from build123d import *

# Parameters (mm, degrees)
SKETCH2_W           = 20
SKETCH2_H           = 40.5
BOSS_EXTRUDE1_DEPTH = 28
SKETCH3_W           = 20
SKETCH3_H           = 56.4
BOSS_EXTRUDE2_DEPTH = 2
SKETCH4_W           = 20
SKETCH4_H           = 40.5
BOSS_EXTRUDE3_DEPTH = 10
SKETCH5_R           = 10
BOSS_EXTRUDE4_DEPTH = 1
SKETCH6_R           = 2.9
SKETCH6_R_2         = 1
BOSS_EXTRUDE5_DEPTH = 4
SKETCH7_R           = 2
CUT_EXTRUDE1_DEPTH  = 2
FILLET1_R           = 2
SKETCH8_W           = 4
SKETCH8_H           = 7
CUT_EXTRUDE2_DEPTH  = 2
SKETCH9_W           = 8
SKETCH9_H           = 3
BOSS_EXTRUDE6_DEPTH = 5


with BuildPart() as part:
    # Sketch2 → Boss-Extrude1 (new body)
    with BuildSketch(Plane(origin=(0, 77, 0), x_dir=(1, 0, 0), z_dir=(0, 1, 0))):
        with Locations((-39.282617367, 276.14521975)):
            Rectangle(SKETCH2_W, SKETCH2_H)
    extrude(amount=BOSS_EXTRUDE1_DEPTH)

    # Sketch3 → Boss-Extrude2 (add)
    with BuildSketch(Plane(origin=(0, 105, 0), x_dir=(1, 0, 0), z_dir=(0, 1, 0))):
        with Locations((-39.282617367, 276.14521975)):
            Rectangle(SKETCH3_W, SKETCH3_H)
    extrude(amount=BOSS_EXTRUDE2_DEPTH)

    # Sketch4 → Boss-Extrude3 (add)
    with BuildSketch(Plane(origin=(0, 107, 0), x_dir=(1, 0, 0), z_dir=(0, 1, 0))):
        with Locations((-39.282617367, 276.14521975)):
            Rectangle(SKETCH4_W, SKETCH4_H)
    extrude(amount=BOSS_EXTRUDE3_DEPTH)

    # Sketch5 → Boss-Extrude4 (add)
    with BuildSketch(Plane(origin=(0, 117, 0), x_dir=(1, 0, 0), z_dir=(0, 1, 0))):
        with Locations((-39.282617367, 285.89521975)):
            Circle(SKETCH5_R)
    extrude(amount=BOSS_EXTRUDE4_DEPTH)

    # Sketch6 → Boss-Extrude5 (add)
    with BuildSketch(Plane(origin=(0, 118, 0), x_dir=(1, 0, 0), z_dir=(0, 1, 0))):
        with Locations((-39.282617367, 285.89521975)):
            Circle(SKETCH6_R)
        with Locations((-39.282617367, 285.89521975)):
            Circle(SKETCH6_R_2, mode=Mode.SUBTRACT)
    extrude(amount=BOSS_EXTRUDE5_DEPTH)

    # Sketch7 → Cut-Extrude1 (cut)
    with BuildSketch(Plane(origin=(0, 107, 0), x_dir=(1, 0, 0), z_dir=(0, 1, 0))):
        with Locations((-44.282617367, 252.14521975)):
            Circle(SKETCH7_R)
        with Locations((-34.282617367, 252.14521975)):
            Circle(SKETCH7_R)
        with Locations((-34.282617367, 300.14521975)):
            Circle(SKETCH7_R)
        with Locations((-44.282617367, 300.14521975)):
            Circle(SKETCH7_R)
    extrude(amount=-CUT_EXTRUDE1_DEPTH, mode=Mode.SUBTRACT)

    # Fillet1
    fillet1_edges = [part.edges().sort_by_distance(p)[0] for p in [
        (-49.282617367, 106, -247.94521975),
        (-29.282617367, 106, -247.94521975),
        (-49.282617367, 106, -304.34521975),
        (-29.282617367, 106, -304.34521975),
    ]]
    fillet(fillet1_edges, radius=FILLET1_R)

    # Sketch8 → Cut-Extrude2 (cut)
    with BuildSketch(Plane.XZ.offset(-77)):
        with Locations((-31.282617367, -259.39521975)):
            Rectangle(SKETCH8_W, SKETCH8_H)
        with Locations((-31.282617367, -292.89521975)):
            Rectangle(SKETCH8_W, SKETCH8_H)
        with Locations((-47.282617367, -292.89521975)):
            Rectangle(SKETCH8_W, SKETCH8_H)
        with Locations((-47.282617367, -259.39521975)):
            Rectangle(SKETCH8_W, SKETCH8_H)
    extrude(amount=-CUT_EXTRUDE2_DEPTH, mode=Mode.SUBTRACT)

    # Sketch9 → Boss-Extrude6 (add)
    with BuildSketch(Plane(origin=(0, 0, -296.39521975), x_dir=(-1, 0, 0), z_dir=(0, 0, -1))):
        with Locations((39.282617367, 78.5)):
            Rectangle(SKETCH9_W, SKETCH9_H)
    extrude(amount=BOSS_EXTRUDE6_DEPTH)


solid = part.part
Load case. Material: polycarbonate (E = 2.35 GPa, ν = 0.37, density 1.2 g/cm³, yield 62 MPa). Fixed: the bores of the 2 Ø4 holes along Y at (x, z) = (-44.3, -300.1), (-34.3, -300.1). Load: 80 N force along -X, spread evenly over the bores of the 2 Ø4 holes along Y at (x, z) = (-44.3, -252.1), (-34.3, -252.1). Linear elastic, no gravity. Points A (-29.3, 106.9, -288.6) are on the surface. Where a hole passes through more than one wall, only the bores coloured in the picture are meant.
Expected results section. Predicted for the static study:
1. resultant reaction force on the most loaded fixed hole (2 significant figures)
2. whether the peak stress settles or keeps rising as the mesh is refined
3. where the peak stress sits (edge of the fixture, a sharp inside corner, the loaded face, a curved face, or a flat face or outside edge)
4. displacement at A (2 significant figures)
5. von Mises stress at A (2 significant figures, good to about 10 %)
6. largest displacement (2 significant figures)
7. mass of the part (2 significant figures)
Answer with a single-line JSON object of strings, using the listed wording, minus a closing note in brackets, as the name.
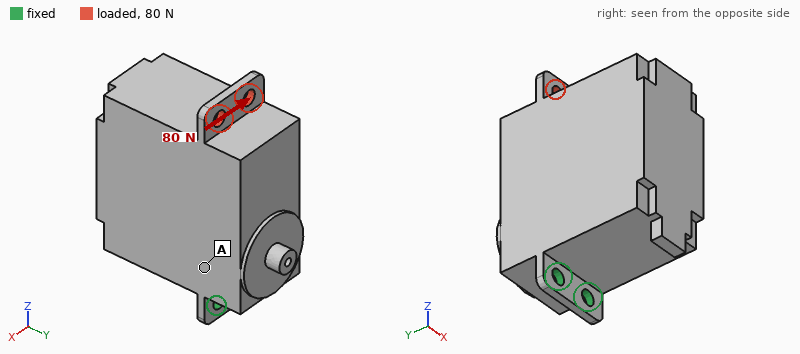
{"resultant reaction force on the most loaded fixed hole": "310 N", "whether the peak stress settles or keeps rising as the mesh is refined": "keeps rising", "where the peak stress sits": "edge of the fixture", "displacement at A": "0.11 mm", "von Mises stress at A": "3.6 MPa", "largest displacement": "0.47 mm", "mass of the part": "40 g"}
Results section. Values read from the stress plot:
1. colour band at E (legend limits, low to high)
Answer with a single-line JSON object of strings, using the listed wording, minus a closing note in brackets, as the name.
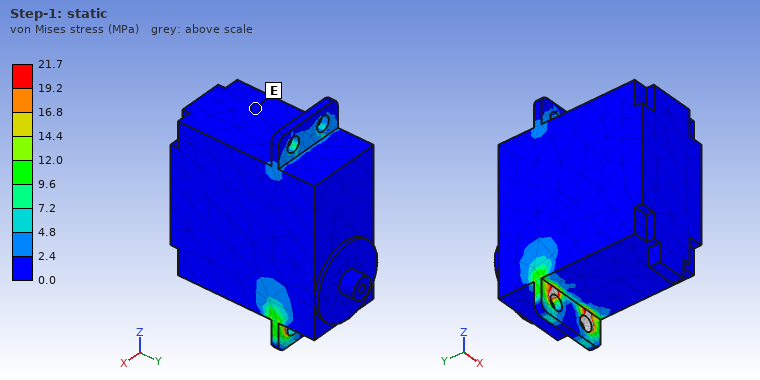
{"colour band at E": "0.0 to 2.4 MPa"}
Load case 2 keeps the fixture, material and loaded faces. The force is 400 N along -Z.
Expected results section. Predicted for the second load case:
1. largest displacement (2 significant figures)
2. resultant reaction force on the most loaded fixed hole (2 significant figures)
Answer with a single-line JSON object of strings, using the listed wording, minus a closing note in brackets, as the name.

{"largest displacement": "95 µm", "resultant reaction force on the most loaded fixed hole": "200 N"}
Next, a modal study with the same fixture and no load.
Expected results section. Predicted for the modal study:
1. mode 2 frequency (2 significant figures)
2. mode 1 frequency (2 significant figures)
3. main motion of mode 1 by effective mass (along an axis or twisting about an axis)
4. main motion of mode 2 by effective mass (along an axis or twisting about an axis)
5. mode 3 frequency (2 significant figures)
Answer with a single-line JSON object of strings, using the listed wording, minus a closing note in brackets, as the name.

{"mode 2 frequency": "530 Hz", "mode 1 frequency": "95 Hz", "main motion of mode 1 by effective mass": "along Y", "main motion of mode 2 by effective mass": "along X", "mode 3 frequency": "880 Hz"}
